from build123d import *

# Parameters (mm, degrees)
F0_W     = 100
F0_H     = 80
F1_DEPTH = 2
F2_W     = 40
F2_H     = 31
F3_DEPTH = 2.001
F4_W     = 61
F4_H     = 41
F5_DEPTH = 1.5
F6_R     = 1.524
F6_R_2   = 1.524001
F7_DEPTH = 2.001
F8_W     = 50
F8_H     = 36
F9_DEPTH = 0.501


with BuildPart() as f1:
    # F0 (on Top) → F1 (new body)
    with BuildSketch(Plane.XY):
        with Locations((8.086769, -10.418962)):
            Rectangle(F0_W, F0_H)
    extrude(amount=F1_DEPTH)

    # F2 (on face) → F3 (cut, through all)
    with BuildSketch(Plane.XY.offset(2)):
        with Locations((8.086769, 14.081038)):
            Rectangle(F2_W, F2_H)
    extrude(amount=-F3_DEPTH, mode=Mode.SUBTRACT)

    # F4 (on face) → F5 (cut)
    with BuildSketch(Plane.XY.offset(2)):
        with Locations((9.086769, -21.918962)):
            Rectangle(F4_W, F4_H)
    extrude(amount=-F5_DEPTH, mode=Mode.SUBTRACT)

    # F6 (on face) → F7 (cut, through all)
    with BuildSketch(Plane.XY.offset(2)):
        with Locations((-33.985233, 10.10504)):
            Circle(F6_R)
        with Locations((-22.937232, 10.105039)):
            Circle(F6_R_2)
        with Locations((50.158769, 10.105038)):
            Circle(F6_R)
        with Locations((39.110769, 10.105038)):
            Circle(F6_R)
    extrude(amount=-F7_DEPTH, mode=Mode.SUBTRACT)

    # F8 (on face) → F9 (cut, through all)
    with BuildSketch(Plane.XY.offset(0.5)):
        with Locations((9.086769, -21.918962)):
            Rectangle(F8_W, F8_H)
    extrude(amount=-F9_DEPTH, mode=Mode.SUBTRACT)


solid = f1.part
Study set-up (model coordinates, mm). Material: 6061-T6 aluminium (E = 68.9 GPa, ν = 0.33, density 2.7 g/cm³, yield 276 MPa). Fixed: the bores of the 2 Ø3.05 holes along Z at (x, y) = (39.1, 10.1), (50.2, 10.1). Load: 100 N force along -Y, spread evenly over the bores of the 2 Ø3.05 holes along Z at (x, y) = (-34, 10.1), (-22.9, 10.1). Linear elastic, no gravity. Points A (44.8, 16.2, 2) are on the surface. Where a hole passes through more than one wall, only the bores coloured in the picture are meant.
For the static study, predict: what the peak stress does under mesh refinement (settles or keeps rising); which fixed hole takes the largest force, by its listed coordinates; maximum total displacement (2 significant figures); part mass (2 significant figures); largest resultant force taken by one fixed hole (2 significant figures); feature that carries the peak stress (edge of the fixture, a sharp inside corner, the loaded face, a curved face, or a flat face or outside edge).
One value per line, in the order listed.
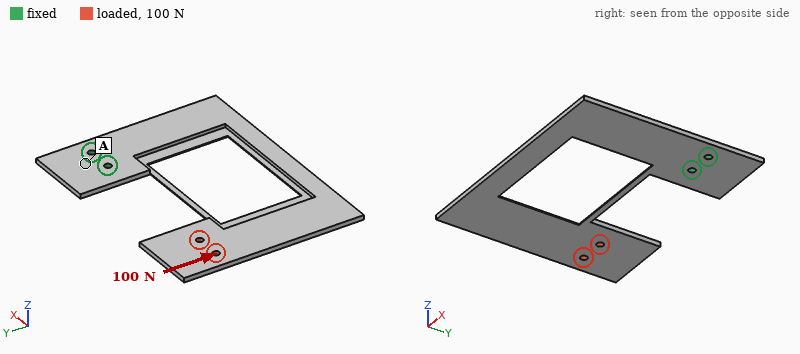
keeps rising
(39.1, 10.1)
1.4 mm
24 g
630 N
a sharp inside corner
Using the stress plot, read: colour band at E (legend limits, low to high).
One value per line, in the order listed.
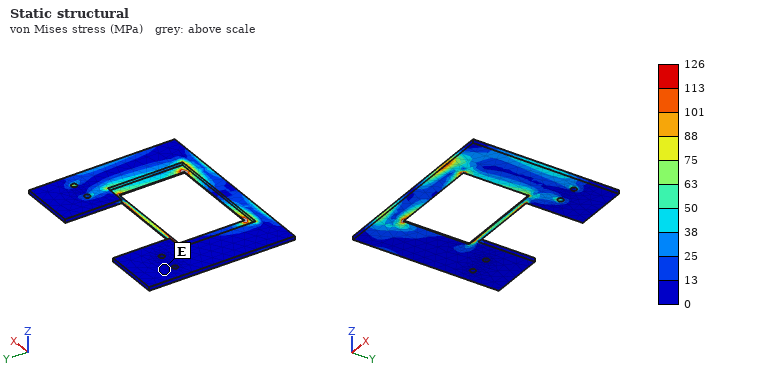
0 to 13 MPa
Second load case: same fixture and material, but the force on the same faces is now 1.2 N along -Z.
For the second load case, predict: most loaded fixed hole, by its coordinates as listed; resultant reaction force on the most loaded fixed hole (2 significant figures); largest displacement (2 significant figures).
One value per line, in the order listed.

(39.1, 10.1)
6.2 N
1.5 mm
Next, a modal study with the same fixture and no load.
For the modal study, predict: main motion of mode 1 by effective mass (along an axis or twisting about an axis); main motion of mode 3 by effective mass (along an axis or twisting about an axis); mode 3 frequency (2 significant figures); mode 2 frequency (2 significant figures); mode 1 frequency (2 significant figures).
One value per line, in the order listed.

along Z
along Z
410 Hz
140 Hz
56 Hz
